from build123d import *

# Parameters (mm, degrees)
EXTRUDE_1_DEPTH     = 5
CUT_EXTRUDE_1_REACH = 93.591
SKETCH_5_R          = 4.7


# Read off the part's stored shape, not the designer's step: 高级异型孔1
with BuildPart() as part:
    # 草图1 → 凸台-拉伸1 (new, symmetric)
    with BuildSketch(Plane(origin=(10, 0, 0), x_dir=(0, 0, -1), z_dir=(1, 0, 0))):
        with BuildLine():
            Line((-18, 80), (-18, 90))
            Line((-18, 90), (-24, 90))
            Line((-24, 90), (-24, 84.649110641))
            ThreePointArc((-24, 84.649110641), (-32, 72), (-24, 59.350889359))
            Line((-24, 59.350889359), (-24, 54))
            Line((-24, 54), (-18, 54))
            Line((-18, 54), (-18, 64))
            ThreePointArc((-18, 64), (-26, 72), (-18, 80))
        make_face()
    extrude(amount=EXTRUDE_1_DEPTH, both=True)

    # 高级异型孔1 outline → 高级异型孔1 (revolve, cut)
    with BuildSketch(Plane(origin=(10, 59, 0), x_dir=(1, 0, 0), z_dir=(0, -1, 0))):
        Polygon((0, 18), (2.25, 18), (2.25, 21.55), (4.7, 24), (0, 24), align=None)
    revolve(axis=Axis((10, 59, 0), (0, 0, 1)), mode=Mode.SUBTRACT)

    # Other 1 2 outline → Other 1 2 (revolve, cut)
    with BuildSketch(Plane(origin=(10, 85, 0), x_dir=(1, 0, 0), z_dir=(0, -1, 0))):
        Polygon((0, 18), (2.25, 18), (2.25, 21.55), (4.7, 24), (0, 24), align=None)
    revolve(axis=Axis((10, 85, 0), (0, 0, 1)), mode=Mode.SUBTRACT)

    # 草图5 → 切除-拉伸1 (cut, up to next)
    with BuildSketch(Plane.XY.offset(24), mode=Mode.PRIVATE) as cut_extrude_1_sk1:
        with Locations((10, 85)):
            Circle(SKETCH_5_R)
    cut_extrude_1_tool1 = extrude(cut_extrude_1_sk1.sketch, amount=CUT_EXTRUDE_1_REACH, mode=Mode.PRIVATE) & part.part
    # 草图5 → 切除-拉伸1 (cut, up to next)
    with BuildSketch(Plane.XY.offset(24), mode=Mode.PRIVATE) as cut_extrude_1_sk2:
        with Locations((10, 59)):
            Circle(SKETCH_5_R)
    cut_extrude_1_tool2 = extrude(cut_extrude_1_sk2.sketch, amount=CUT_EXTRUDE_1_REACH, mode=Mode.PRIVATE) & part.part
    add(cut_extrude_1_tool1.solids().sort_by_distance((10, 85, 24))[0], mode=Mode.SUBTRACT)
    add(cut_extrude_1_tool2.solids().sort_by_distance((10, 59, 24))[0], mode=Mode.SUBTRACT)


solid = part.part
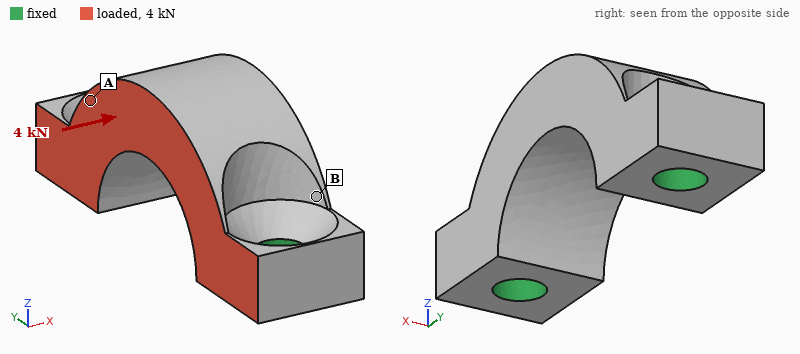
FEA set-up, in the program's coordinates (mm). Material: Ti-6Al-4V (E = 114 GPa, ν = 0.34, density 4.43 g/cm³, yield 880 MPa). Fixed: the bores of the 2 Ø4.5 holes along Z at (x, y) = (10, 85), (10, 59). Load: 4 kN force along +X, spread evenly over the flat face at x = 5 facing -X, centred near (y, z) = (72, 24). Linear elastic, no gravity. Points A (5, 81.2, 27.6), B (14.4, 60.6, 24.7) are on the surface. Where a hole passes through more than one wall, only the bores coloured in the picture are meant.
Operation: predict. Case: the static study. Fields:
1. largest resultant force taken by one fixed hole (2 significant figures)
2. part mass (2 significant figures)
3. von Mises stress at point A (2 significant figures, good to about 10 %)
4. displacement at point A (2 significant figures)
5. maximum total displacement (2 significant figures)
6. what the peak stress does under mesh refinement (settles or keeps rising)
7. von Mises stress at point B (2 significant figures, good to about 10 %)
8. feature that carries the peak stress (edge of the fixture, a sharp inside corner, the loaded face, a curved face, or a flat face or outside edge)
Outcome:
2.0 kN
9.4 g
58 MPa
30 µm
44 µm
keeps rising
140 MPa
edge of the fixture
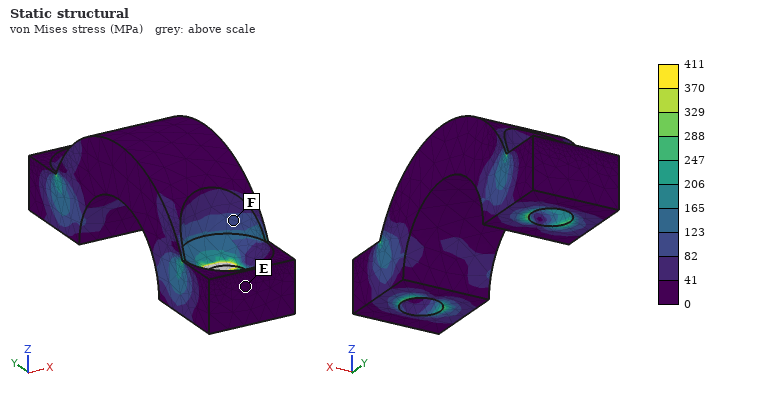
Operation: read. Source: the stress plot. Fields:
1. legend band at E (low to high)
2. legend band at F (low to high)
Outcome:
0 to 41 MPa
82 to 123 MPa
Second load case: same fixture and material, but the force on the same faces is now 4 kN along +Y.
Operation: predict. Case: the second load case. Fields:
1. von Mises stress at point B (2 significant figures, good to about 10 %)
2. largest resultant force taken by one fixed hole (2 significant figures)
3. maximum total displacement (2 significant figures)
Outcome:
59 MPa
2.1 kN
18 µm
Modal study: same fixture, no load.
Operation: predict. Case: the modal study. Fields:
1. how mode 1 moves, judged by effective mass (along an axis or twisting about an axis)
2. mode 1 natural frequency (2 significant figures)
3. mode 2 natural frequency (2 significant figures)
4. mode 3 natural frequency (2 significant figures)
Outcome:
along X
18 kHz
40 kHz
41 kHz
